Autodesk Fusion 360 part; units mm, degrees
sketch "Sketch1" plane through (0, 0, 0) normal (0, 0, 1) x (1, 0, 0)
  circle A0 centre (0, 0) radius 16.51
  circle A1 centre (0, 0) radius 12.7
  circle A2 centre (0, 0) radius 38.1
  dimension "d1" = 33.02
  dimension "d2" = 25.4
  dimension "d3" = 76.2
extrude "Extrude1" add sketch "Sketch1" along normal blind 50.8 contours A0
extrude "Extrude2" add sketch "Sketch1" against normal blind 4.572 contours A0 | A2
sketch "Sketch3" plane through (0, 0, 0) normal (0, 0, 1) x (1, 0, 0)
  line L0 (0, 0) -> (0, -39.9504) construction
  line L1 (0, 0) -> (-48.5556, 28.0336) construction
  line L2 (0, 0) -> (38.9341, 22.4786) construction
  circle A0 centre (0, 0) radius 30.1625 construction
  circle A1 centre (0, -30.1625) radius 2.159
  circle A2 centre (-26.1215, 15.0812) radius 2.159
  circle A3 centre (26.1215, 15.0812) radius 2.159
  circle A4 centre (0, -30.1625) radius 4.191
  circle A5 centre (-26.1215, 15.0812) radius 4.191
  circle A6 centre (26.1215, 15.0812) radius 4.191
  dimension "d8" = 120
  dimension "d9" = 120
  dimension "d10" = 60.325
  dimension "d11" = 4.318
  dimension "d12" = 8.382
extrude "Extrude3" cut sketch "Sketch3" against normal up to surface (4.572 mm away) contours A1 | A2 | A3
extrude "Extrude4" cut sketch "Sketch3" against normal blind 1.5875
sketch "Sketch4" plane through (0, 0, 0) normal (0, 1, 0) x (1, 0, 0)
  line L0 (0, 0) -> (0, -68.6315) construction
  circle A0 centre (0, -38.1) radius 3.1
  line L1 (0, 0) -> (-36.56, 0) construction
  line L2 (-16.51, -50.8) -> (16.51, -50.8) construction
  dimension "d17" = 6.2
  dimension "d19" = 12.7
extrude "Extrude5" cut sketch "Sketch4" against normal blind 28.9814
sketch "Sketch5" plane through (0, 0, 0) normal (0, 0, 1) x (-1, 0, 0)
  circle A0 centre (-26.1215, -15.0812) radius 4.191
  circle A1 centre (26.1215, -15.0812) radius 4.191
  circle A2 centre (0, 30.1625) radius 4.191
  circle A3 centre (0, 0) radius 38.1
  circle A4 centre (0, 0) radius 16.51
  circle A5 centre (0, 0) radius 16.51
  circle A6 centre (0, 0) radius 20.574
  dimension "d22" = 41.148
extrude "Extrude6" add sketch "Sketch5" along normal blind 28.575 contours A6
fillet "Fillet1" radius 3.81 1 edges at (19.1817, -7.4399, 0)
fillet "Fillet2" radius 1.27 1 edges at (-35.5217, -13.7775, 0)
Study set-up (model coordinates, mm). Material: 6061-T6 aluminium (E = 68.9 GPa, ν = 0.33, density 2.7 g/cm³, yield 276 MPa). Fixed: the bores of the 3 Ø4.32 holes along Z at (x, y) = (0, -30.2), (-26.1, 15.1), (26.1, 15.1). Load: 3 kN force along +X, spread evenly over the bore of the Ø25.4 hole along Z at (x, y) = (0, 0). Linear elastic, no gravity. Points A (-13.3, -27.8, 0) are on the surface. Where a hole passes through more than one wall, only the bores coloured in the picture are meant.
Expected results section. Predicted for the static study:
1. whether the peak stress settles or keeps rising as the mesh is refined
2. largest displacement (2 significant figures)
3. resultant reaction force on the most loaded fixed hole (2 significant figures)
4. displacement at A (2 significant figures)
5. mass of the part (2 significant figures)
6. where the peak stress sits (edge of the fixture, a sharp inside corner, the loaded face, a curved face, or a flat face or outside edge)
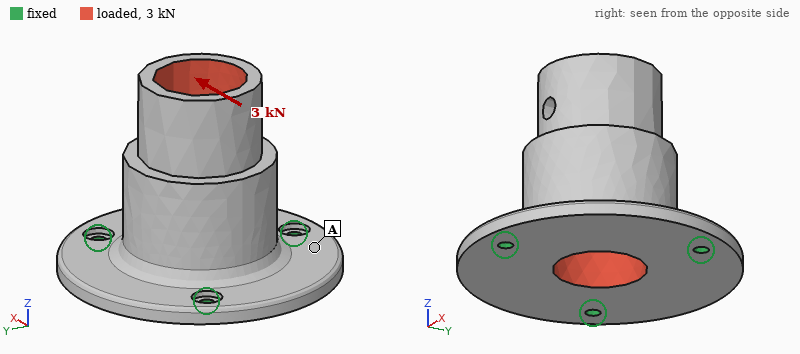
keeps rising
85 µm
2.1 kN
18 µm
130 g
edge of the fixture
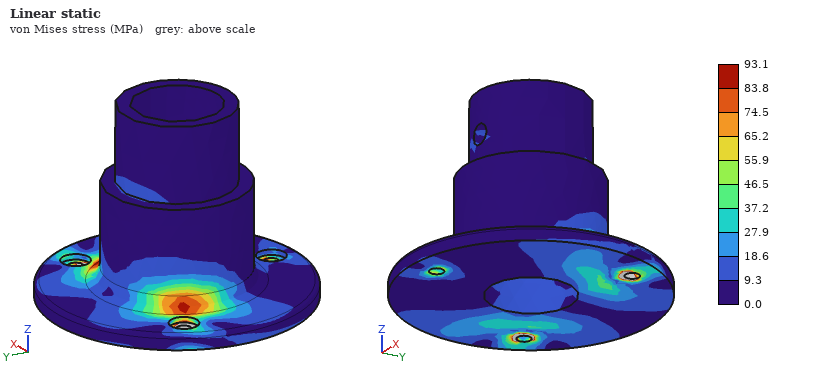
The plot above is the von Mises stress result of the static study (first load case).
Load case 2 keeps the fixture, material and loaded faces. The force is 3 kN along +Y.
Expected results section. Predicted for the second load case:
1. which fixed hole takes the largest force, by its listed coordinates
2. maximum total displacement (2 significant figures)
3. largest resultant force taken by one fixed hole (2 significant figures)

(0, -30.2)
85 µm
2.5 kN
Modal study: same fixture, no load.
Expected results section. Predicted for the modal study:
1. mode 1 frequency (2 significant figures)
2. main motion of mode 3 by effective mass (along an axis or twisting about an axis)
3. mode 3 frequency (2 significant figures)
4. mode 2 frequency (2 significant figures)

4000 Hz
along Z
5700 Hz
4000 Hz
